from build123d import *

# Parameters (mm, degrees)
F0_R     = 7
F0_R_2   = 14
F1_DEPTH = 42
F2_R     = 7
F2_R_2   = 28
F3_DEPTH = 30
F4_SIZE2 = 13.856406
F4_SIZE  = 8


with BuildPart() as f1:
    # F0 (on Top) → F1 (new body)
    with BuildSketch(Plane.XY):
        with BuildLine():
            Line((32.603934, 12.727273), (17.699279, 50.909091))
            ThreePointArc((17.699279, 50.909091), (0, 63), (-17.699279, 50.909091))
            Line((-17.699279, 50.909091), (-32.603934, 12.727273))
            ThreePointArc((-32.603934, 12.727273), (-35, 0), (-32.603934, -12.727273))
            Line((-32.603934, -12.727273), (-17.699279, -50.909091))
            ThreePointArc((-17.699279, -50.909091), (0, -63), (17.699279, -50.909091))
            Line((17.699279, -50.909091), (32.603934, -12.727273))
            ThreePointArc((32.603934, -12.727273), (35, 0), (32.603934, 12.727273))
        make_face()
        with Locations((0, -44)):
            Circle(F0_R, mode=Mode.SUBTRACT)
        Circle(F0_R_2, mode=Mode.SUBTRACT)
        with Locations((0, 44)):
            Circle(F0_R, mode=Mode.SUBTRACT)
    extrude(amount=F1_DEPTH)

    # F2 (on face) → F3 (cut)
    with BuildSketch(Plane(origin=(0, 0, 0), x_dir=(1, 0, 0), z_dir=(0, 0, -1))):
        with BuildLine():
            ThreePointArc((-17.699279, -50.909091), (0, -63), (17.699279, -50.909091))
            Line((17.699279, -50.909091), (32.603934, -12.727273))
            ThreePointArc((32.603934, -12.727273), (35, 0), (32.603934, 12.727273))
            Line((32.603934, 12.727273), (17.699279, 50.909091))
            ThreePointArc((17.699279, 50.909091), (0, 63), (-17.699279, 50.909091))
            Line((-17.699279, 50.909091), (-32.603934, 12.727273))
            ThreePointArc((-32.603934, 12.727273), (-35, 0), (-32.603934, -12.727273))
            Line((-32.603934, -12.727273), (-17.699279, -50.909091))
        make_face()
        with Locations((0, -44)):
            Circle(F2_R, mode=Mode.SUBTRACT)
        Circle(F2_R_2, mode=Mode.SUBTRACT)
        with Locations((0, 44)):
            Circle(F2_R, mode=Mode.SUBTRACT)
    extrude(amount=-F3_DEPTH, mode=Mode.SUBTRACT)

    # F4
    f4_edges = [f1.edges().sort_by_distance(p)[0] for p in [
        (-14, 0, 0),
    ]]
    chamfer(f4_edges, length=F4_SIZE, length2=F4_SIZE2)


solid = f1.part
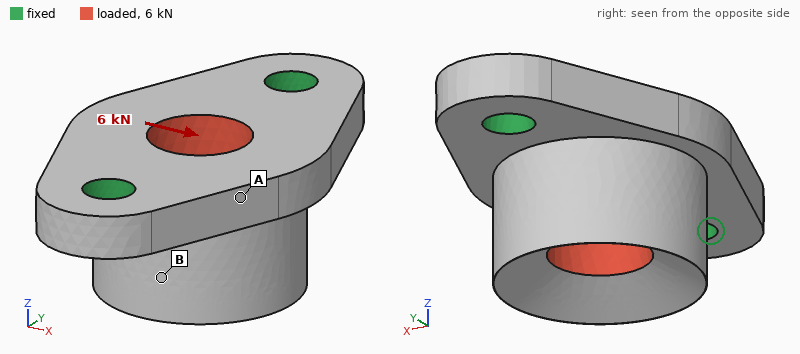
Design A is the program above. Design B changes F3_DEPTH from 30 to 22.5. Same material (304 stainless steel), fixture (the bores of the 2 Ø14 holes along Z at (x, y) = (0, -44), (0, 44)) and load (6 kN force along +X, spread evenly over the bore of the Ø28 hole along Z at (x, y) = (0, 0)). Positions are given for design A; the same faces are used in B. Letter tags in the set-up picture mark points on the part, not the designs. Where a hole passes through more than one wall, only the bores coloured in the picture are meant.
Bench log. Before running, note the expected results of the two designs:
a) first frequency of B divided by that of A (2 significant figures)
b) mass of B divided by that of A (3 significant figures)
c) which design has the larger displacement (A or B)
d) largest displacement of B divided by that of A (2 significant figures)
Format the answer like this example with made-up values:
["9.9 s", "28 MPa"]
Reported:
["1.7", "1.23", "A", "0.28"]
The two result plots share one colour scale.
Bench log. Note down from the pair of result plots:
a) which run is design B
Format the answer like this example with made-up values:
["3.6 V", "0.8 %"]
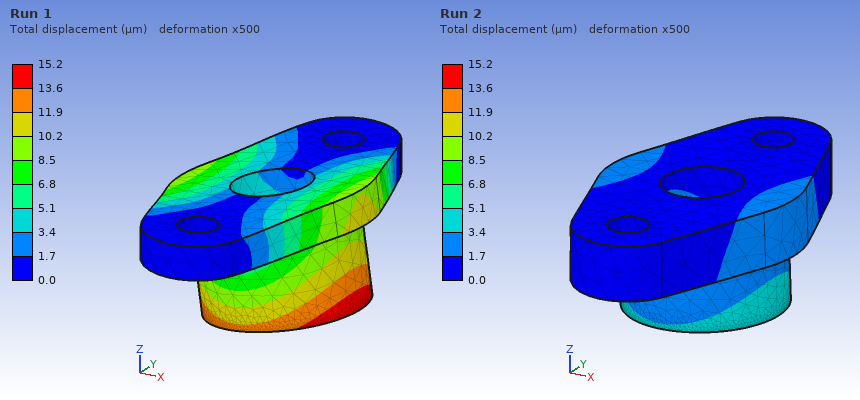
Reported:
["Run 2"]
